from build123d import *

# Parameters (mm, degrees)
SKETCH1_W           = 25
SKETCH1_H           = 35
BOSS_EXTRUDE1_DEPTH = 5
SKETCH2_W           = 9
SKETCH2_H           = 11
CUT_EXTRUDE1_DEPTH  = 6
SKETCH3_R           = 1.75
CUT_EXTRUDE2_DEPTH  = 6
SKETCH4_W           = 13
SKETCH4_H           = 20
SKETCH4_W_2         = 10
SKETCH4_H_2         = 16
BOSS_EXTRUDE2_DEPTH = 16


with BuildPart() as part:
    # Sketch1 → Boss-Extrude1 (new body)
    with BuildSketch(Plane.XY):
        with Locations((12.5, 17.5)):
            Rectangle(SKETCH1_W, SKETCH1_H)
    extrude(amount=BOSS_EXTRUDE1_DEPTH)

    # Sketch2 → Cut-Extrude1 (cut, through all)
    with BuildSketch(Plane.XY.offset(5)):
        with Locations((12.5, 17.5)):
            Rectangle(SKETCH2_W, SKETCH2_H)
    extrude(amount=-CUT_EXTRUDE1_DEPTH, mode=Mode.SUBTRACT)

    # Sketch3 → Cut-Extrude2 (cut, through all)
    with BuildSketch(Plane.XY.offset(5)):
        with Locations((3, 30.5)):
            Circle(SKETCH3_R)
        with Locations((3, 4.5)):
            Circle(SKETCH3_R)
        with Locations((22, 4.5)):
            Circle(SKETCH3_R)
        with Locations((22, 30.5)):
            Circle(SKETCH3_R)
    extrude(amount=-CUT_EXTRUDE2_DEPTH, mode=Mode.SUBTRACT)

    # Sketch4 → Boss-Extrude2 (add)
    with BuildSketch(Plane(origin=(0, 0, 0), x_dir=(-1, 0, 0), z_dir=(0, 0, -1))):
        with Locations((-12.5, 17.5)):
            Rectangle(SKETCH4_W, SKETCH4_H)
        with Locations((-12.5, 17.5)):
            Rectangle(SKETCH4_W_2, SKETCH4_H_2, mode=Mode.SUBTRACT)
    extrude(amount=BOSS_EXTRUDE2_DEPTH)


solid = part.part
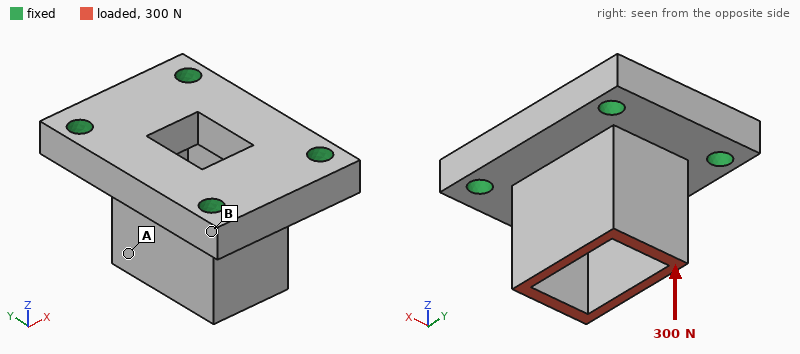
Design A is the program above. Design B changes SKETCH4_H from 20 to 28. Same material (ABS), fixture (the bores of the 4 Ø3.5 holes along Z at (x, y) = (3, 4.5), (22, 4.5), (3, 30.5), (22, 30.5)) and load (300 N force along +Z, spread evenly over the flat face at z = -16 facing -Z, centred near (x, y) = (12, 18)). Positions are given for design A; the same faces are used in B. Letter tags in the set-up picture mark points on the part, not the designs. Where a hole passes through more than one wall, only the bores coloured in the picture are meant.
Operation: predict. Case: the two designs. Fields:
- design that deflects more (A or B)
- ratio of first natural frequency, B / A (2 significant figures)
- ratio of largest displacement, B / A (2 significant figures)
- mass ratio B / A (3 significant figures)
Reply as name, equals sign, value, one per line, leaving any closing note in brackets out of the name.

design that deflects more = A
ratio of first natural frequency, B / A = 1.1
ratio of largest displacement, B / A = 0.51
mass ratio B / A = 1.31
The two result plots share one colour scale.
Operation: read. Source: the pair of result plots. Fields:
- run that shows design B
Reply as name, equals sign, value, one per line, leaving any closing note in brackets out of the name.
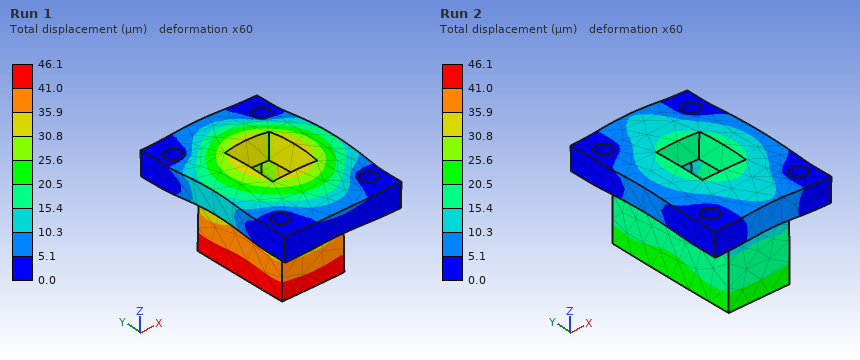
run that shows design B = Run 2
